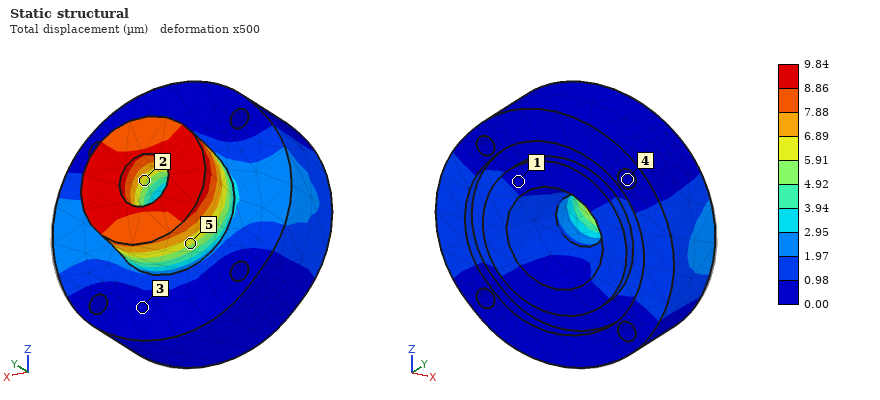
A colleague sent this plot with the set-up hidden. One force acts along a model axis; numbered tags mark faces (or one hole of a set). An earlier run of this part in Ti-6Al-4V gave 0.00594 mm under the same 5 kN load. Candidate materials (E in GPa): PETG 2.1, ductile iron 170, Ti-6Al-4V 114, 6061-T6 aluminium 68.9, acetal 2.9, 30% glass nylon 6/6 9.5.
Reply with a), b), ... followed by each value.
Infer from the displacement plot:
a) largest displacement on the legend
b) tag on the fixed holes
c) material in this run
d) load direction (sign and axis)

a) 9.84 µm
b) 4
c) 6061-T6 aluminium
d) -X
